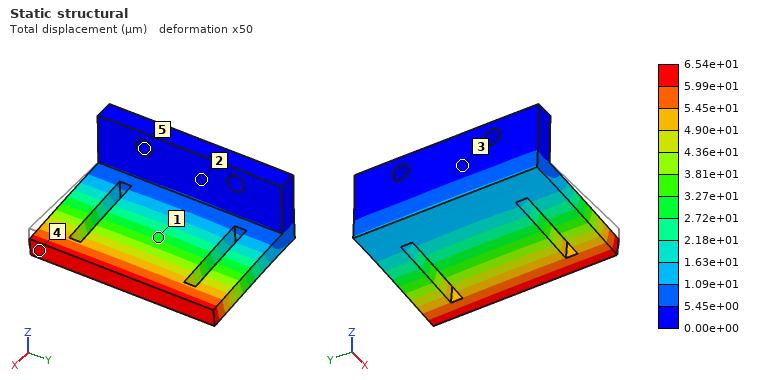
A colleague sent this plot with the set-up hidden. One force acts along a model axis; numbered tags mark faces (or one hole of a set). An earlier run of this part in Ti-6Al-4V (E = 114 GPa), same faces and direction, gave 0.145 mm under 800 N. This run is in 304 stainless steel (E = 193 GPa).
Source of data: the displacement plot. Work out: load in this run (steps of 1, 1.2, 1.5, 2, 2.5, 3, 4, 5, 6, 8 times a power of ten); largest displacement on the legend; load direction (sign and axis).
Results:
600 N
6.54e+01 µm
-Z
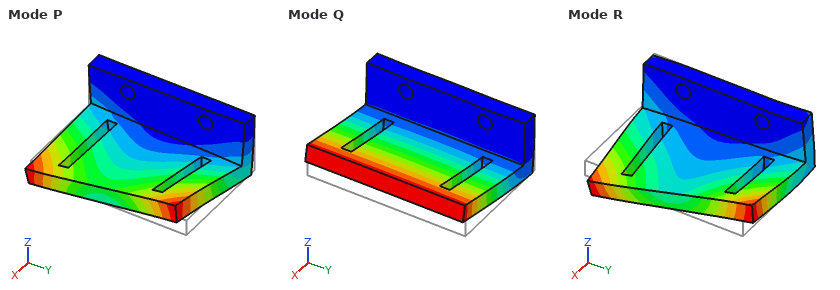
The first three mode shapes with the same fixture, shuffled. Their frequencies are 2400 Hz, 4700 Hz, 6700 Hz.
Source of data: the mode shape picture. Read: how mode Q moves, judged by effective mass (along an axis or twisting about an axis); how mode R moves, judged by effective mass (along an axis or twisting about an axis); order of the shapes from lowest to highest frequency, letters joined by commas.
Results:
along Z
along Y
Q, P, R
